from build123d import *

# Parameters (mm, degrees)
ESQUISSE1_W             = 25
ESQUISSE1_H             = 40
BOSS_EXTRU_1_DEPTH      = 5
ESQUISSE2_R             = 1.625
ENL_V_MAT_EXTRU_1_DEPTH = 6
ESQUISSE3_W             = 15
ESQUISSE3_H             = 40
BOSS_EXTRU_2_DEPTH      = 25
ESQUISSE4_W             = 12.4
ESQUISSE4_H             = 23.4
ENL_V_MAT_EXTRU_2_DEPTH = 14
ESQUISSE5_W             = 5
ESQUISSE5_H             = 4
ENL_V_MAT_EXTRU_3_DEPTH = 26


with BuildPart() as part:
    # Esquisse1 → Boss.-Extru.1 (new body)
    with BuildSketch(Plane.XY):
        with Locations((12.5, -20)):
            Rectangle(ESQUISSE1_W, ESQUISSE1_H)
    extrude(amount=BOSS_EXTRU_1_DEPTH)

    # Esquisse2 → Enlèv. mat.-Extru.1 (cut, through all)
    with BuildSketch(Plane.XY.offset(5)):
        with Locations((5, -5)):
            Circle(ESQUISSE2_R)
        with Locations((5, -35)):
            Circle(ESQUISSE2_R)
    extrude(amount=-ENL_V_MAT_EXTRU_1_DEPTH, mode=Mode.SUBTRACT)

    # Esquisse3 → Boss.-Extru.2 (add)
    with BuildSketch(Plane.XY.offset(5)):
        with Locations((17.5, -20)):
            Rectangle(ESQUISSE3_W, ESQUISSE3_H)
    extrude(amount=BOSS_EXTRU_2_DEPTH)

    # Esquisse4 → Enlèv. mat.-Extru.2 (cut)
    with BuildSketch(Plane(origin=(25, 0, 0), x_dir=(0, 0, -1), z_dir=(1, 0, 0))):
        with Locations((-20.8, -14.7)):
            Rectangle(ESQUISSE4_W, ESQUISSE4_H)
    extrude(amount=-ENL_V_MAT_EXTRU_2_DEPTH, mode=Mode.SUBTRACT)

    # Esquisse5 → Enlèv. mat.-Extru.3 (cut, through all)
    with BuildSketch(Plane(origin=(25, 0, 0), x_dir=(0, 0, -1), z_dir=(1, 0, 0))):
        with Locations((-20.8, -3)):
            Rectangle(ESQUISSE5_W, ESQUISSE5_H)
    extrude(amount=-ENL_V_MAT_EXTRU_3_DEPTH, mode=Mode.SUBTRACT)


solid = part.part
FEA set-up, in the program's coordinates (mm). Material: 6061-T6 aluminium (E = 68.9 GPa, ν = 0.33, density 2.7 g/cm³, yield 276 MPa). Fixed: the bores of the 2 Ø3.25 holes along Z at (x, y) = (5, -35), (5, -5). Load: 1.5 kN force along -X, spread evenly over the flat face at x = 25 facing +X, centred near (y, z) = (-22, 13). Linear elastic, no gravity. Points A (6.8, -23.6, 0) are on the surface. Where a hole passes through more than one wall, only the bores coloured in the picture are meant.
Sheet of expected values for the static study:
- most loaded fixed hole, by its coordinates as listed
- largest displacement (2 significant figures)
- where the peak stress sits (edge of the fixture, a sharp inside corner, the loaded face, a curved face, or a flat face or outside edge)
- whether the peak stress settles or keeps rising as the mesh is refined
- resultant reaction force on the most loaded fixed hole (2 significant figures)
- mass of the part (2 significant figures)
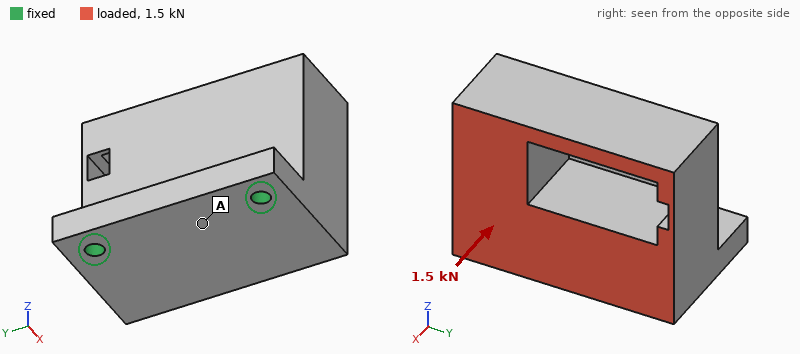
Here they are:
(5, -35)
0.18 mm
edge of the fixture
keeps rising
850 N
42 g
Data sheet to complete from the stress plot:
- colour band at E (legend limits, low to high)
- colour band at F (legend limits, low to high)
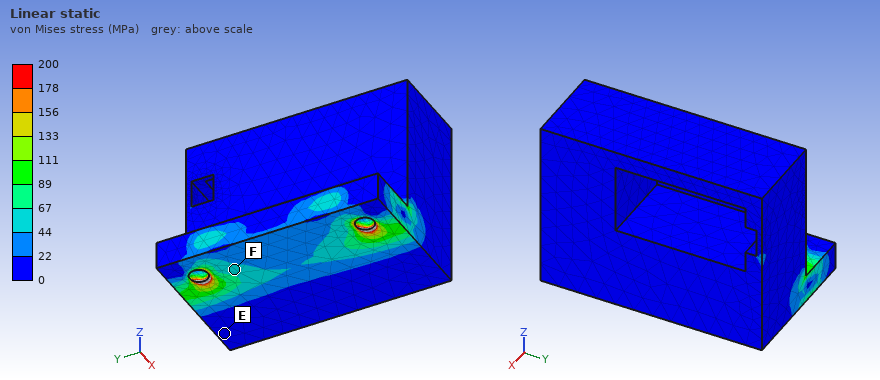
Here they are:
0 to 22 MPa
44 to 67 MPa
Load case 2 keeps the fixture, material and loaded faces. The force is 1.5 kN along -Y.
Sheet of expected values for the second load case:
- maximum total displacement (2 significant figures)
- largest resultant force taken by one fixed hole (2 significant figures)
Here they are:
22 µm
1.3 kN
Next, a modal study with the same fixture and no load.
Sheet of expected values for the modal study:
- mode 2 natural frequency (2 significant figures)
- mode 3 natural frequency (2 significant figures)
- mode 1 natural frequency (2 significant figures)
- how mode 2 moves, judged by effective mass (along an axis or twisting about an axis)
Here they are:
8100 Hz
12 kHz
2500 Hz
along Y
